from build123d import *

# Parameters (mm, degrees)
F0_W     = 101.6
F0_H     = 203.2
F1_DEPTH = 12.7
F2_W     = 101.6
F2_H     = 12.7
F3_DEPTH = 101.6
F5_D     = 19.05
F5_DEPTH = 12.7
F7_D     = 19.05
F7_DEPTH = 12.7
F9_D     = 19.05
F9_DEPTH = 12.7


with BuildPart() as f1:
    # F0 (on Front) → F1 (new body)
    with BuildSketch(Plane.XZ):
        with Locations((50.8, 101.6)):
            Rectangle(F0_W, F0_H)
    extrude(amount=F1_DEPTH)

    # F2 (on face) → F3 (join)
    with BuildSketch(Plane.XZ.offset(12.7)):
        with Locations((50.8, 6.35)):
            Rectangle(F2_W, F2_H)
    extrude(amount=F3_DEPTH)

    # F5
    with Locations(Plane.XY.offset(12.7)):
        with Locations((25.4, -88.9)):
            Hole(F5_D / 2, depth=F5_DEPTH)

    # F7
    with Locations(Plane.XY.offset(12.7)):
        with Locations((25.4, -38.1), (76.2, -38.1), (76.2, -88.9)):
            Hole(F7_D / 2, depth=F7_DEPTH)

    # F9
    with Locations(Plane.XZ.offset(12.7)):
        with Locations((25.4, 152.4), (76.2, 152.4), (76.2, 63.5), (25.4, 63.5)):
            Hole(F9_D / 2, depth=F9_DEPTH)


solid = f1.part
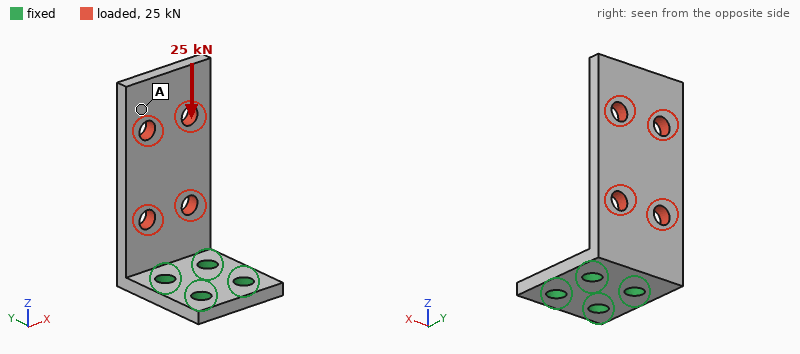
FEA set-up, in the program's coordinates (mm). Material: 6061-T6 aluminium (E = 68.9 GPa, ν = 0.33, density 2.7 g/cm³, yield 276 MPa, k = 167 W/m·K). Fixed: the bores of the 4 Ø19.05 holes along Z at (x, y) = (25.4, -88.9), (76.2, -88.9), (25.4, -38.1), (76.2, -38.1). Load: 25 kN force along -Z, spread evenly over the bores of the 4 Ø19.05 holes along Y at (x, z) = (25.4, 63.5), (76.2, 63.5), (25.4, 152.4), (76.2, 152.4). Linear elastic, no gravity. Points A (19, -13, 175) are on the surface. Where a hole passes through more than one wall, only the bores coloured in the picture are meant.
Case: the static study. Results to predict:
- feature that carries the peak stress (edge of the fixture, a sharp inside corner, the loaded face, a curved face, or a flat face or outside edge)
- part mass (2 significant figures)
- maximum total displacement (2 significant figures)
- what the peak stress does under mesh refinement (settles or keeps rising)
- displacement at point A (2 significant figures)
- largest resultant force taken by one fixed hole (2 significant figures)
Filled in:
edge of the fixture
980 g
1.4 mm
keeps rising
1.2 mm
13 kN
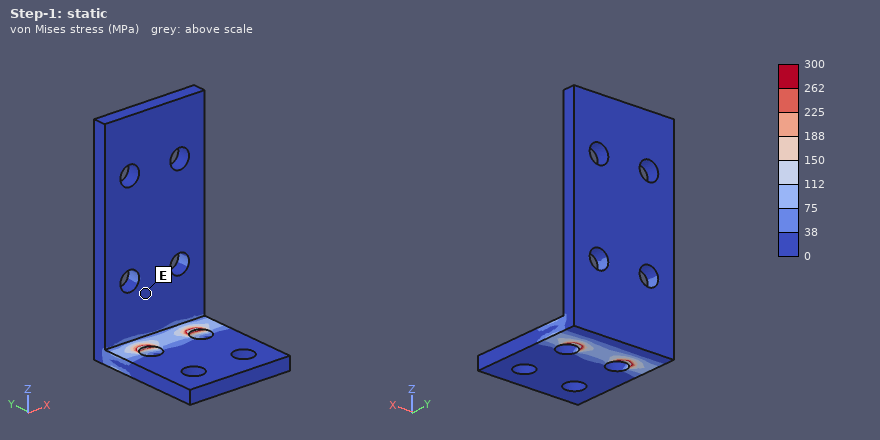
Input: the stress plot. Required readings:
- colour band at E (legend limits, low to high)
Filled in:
0 to 38 MPa
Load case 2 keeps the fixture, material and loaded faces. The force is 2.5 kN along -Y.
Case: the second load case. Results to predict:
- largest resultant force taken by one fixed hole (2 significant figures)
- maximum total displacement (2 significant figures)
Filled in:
1.4 kN
2.9 mm
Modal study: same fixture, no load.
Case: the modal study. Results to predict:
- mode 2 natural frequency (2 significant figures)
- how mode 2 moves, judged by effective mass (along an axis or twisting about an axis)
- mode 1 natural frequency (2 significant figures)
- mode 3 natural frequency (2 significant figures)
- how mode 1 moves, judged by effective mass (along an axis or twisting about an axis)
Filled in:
760 Hz
along X
230 Hz
1000 Hz
along Y
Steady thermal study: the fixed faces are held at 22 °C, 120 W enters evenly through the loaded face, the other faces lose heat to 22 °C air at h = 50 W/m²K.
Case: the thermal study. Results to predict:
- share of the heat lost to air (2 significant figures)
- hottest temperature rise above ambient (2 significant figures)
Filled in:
50 %
37 K
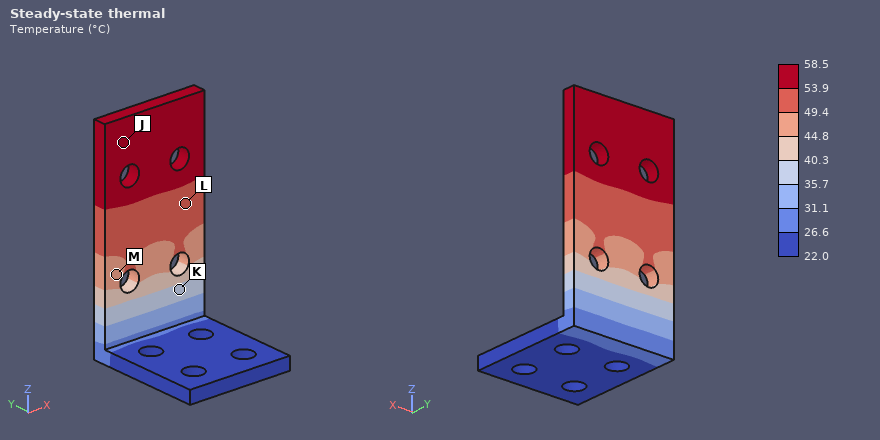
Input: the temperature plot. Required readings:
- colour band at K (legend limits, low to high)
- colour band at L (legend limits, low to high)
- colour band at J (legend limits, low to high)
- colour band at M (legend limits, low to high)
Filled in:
35.7 to 40.3 °C
49.4 to 53.9 °C
53.9 to 58.5 °C
44.8 to 49.4 °C
